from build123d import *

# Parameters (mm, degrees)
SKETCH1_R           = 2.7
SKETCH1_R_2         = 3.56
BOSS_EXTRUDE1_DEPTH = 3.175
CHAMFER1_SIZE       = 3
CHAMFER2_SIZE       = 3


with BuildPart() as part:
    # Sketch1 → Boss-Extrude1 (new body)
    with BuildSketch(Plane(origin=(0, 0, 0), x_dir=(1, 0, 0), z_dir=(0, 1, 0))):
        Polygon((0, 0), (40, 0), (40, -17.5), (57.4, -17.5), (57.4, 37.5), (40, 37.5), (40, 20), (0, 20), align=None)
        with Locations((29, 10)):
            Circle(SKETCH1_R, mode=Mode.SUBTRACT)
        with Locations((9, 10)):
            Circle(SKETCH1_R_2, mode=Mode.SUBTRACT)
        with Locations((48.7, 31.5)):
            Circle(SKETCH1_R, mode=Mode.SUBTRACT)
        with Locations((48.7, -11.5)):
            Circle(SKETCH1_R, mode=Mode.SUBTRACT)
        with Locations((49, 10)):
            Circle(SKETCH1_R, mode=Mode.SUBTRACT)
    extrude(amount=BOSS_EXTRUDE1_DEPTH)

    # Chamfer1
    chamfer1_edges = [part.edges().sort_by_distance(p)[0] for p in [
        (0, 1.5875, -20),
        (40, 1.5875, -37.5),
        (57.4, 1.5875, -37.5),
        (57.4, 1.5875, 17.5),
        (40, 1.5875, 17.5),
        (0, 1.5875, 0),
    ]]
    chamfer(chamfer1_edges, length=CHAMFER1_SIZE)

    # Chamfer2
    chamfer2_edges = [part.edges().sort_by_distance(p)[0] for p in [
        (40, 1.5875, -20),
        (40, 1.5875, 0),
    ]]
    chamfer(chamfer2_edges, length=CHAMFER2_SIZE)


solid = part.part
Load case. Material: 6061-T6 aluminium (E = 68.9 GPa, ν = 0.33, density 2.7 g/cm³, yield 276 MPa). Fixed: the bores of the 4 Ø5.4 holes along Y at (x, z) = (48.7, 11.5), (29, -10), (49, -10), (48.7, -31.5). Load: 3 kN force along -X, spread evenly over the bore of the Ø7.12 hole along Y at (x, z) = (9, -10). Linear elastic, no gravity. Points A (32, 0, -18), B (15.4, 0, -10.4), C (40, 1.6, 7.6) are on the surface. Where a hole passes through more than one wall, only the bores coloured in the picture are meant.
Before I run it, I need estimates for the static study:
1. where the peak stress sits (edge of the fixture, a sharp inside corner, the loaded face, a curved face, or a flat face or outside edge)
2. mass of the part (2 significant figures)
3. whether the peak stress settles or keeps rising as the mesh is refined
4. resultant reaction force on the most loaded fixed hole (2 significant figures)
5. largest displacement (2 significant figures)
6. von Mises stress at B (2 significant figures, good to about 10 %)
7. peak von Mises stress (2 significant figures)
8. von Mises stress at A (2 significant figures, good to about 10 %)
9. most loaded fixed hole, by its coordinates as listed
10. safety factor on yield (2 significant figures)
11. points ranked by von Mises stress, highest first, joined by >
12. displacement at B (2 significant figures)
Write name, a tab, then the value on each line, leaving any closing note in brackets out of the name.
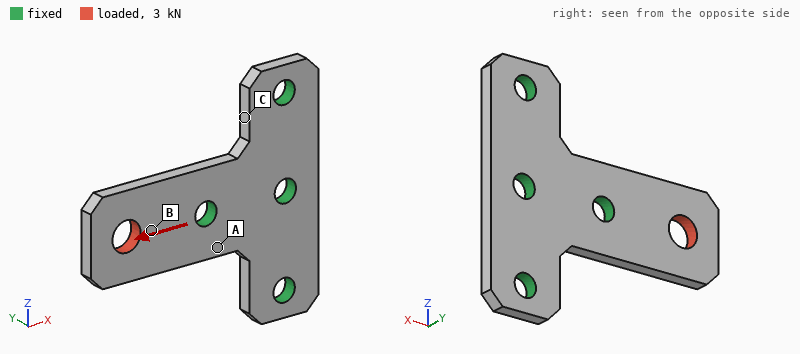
where the peak stress sits	the loaded face
mass of the part	14 g
whether the peak stress settles or keeps rising as the mesh is refined	settles
resultant reaction force on the most loaded fixed hole	2.5 kN
largest displacement	25 µm
von Mises stress at B	55 MPa
peak von Mises stress	130 MPa
von Mises stress at A	23 MPa
most loaded fixed hole, by its coordinates as listed	(29, -10)
safety factor on yield	2.1
points ranked by von Mises stress, highest first, joined by >	B > A > C
displacement at B	10 µm
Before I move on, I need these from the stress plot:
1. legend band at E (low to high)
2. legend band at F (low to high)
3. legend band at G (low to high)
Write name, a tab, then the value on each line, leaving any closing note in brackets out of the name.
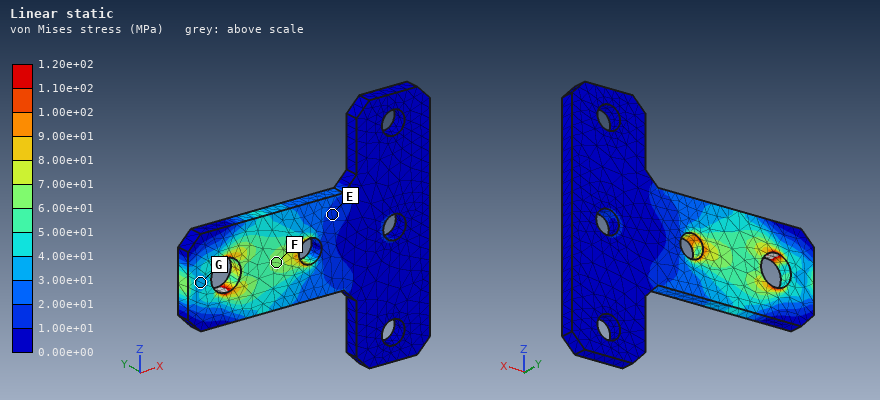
legend band at E	1.00e+01 to 2.00e+01 MPa
legend band at F	6.00e+01 to 7.00e+01 MPa
legend band at G	3.00e+01 to 4.00e+01 MPa
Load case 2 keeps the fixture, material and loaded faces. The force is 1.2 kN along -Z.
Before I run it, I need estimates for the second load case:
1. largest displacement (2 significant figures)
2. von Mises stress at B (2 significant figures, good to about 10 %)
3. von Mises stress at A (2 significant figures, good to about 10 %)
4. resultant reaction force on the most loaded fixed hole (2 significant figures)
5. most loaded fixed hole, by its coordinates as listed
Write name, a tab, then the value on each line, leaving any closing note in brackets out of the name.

largest displacement	93 µm
von Mises stress at B	67 MPa
von Mises stress at A	57 MPa
resultant reaction force on the most loaded fixed hole	1.8 kN
most loaded fixed hole, by its coordinates as listed	(29, -10)
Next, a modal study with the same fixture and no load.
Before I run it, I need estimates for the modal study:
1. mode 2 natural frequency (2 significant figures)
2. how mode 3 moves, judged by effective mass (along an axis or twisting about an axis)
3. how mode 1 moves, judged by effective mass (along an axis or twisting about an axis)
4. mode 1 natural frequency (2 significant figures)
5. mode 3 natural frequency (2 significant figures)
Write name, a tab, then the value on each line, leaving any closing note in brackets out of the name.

mode 2 natural frequency	8800 Hz
how mode 3 moves, judged by effective mass	along Z
how mode 1 moves, judged by effective mass	along Y
mode 1 natural frequency	3600 Hz
mode 3 natural frequency	12 kHz
